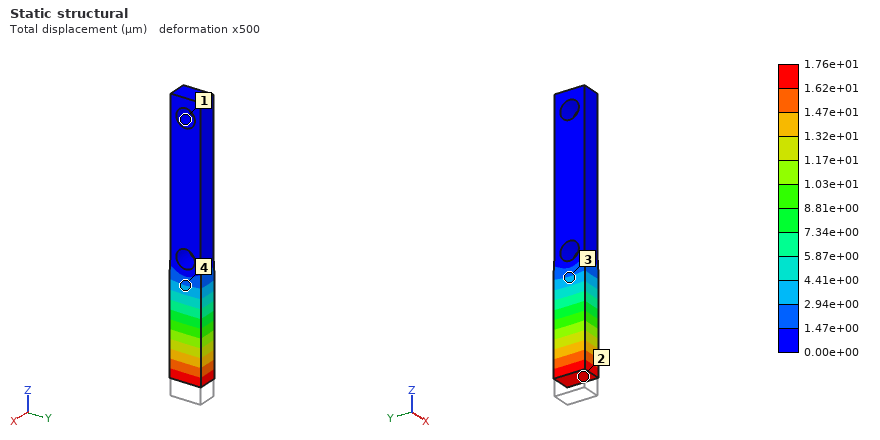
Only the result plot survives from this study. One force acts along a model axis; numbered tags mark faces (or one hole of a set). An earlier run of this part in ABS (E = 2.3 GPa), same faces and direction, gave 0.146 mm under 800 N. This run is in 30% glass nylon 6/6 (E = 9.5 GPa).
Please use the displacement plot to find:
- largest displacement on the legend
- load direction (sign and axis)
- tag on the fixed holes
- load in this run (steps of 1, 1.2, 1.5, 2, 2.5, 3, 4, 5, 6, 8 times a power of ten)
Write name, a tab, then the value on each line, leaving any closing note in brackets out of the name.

largest displacement on the legend	1.76e+01 µm
load direction	+Z
tag on the fixed holes	1
load in this run	400 N
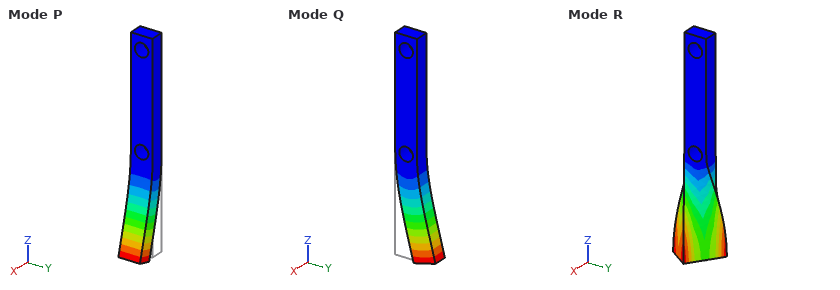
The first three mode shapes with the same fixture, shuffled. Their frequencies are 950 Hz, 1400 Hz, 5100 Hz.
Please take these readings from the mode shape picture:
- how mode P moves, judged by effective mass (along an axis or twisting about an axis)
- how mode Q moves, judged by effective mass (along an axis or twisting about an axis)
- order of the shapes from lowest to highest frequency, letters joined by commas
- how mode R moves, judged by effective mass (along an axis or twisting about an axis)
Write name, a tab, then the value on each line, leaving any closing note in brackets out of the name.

how mode P moves, judged by effective mass	along X
how mode Q moves, judged by effective mass	along Y
order of the shapes from lowest to highest frequency, letters joined by commas	P, Q, R
how mode R moves, judged by effective mass	twisting about Z
